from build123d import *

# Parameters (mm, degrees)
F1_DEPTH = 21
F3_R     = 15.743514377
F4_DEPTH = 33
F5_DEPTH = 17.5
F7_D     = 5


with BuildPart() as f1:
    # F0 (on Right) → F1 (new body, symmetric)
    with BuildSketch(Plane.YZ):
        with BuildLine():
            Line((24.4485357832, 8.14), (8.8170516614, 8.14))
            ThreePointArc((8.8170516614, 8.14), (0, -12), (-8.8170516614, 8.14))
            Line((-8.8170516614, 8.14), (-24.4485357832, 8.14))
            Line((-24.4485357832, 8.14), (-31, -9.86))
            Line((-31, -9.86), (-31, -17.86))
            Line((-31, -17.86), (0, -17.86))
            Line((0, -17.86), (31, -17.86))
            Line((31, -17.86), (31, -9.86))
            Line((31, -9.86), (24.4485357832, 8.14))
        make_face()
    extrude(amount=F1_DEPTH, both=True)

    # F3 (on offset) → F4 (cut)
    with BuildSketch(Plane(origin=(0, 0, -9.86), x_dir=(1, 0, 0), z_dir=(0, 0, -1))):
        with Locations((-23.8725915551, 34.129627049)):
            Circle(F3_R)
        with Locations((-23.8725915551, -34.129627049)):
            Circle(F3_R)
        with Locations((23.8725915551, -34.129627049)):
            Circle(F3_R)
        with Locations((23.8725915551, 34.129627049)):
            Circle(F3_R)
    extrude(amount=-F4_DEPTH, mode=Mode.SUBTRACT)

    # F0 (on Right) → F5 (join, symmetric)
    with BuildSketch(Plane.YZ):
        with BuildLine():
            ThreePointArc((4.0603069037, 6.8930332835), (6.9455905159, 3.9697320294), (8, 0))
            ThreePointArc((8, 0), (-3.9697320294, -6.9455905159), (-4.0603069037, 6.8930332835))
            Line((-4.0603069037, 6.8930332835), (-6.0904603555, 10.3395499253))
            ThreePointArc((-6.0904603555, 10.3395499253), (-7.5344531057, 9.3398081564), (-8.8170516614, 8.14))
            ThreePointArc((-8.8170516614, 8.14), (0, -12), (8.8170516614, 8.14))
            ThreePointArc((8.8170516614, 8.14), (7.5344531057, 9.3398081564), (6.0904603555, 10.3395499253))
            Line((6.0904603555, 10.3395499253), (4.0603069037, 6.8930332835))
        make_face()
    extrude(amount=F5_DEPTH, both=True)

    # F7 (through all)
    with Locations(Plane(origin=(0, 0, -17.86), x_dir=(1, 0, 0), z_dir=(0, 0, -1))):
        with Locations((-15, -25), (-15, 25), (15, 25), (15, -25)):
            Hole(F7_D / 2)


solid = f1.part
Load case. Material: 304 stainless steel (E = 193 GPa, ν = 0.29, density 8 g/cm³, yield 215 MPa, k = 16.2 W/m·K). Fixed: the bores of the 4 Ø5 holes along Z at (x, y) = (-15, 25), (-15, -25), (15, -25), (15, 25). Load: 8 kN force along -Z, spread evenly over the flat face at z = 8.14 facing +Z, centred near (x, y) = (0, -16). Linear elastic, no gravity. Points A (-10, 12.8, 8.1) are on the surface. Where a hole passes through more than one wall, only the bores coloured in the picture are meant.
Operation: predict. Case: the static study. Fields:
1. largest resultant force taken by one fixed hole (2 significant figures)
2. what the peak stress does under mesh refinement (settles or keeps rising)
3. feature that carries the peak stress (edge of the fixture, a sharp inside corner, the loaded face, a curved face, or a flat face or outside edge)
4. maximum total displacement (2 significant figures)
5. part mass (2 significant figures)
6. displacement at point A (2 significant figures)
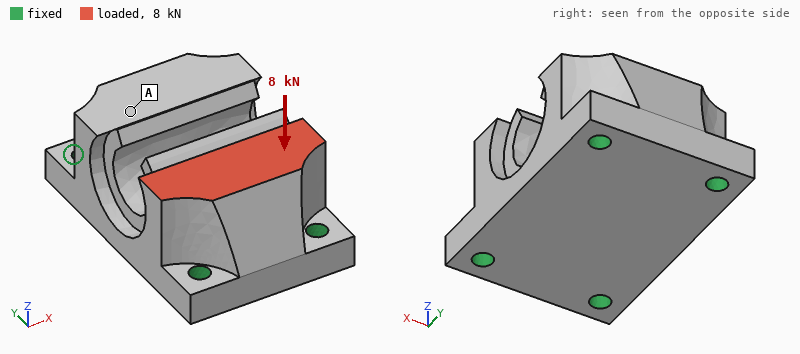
3.5 kN
keeps rising
edge of the fixture
9.1 µm
380 g
4.9 µm
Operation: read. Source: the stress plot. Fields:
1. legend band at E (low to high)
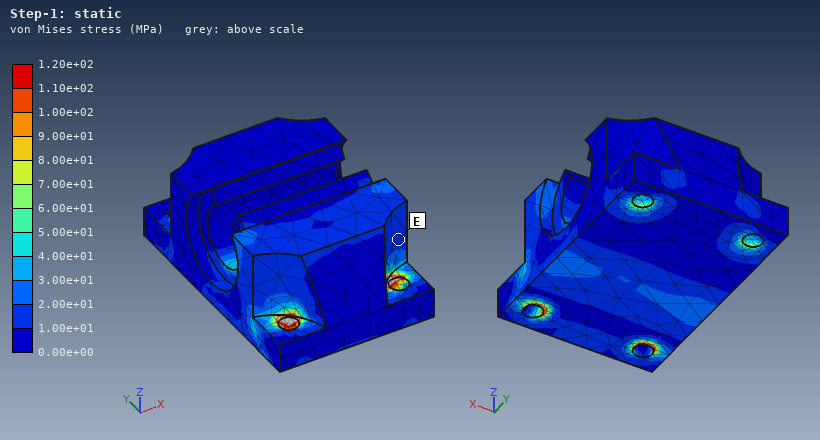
1.00e+01 to 2.00e+01 MPa
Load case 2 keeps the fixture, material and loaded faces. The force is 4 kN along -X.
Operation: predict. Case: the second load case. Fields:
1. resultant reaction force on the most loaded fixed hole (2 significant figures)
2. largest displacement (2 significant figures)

3.1 kN
7.3 µm
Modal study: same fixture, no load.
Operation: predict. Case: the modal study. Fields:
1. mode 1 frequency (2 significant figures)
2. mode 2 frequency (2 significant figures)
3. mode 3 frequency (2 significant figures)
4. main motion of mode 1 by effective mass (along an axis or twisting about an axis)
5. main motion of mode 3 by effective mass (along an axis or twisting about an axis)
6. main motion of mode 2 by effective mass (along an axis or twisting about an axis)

9100 Hz
16 kHz
18 kHz
along Z
along Y
along X
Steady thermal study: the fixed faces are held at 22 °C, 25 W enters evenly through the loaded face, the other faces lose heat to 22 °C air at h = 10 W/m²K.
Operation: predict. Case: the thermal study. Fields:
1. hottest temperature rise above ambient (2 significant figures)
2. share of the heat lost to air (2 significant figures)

74 K
7.6 %
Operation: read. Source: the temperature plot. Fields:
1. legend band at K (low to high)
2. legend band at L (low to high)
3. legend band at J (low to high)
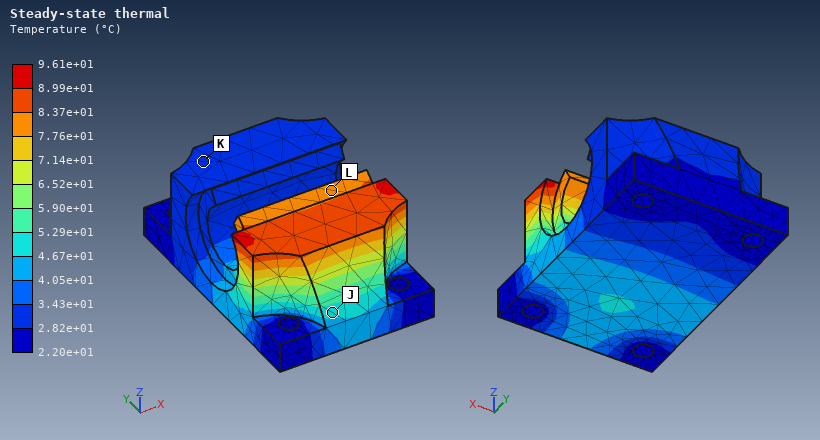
2.82e+01 to 3.43e+01 °C
7.76e+01 to 8.37e+01 °C
4.67e+01 to 5.29e+01 °C
